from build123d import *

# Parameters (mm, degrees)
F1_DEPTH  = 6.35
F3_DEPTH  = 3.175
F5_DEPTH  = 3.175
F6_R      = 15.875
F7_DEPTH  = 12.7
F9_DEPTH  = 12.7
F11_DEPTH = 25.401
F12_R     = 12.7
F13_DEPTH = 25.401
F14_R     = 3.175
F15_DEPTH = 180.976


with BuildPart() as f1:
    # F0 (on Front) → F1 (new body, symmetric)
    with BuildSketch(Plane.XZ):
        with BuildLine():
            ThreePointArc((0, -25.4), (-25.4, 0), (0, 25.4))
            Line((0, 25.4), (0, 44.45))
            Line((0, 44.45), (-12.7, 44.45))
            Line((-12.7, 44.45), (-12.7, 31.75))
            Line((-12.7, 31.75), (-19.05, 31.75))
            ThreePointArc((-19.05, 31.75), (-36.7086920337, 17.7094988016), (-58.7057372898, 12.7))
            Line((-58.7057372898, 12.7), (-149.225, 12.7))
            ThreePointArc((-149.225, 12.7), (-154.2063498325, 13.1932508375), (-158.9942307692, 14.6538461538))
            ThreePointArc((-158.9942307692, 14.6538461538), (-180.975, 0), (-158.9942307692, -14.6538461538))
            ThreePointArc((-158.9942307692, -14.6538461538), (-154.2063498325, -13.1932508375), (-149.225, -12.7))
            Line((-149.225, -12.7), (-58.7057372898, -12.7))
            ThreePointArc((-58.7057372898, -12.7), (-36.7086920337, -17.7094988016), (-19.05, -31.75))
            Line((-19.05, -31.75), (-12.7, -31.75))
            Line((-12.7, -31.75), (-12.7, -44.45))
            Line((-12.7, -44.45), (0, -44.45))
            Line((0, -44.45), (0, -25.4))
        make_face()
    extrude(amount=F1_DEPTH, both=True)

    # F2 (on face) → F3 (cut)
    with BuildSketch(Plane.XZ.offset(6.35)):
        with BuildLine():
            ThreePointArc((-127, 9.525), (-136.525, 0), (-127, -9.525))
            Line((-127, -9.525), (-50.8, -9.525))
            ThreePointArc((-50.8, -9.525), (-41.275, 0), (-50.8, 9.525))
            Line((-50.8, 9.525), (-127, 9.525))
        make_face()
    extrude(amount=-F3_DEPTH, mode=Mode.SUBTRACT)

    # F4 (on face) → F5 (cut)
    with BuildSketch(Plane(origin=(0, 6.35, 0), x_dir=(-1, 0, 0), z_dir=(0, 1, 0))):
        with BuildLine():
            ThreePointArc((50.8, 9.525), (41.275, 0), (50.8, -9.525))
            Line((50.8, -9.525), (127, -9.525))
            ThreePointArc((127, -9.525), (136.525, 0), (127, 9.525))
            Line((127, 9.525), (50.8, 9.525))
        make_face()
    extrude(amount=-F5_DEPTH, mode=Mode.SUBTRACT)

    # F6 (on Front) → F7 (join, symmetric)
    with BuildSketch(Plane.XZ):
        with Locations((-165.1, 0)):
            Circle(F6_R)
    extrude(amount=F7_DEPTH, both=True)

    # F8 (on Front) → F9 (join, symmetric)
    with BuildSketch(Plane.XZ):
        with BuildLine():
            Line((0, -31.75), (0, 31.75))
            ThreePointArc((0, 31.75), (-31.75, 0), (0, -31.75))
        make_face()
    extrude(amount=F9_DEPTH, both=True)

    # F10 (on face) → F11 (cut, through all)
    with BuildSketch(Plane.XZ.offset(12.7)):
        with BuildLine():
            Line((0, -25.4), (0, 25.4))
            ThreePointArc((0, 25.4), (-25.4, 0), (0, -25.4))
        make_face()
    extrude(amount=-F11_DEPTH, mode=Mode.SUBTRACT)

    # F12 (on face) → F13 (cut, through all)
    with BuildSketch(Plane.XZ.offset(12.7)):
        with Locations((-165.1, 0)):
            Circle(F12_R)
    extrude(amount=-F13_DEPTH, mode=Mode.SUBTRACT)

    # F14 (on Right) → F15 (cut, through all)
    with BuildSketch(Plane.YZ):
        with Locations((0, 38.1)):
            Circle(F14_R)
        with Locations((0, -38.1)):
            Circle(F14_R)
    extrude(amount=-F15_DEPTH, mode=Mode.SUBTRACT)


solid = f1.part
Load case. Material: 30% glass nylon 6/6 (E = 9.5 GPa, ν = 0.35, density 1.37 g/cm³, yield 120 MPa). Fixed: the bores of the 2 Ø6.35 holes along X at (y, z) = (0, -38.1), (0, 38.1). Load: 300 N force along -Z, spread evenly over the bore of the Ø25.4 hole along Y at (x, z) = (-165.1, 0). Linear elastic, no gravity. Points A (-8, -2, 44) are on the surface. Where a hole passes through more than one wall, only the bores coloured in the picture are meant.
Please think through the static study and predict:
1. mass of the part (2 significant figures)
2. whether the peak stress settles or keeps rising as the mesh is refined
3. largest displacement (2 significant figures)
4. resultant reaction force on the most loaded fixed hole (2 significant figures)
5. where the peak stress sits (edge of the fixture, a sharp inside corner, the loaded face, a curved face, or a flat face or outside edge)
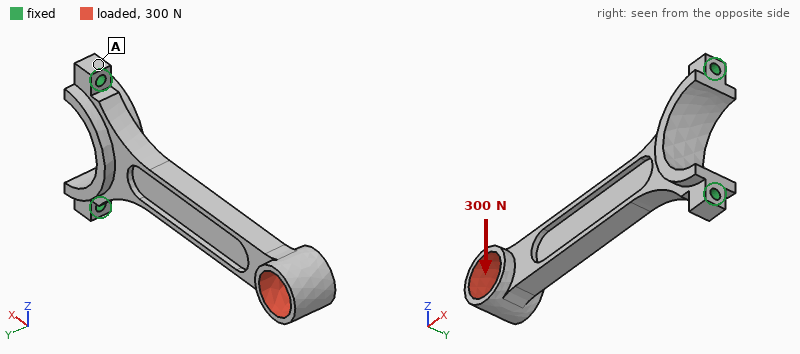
79 g
keeps rising
2.4 mm
860 N
edge of the fixture
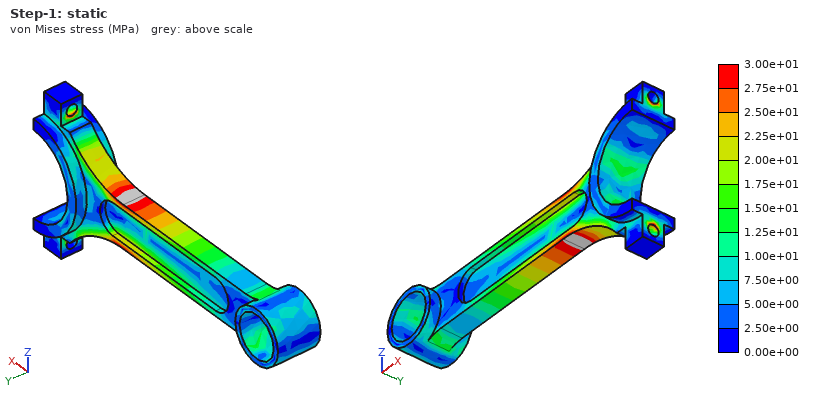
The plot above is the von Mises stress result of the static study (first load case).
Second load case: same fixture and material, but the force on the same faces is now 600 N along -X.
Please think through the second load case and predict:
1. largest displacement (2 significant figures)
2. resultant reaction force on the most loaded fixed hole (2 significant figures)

93 µm
380 N
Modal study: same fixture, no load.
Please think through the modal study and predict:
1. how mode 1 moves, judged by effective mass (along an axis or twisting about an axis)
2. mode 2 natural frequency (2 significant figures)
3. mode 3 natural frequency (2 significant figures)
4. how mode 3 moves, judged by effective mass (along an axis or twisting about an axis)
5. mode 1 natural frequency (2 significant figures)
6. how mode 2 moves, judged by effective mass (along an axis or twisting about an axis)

along Y
470 Hz
880 Hz
along Y
160 Hz
along Z
